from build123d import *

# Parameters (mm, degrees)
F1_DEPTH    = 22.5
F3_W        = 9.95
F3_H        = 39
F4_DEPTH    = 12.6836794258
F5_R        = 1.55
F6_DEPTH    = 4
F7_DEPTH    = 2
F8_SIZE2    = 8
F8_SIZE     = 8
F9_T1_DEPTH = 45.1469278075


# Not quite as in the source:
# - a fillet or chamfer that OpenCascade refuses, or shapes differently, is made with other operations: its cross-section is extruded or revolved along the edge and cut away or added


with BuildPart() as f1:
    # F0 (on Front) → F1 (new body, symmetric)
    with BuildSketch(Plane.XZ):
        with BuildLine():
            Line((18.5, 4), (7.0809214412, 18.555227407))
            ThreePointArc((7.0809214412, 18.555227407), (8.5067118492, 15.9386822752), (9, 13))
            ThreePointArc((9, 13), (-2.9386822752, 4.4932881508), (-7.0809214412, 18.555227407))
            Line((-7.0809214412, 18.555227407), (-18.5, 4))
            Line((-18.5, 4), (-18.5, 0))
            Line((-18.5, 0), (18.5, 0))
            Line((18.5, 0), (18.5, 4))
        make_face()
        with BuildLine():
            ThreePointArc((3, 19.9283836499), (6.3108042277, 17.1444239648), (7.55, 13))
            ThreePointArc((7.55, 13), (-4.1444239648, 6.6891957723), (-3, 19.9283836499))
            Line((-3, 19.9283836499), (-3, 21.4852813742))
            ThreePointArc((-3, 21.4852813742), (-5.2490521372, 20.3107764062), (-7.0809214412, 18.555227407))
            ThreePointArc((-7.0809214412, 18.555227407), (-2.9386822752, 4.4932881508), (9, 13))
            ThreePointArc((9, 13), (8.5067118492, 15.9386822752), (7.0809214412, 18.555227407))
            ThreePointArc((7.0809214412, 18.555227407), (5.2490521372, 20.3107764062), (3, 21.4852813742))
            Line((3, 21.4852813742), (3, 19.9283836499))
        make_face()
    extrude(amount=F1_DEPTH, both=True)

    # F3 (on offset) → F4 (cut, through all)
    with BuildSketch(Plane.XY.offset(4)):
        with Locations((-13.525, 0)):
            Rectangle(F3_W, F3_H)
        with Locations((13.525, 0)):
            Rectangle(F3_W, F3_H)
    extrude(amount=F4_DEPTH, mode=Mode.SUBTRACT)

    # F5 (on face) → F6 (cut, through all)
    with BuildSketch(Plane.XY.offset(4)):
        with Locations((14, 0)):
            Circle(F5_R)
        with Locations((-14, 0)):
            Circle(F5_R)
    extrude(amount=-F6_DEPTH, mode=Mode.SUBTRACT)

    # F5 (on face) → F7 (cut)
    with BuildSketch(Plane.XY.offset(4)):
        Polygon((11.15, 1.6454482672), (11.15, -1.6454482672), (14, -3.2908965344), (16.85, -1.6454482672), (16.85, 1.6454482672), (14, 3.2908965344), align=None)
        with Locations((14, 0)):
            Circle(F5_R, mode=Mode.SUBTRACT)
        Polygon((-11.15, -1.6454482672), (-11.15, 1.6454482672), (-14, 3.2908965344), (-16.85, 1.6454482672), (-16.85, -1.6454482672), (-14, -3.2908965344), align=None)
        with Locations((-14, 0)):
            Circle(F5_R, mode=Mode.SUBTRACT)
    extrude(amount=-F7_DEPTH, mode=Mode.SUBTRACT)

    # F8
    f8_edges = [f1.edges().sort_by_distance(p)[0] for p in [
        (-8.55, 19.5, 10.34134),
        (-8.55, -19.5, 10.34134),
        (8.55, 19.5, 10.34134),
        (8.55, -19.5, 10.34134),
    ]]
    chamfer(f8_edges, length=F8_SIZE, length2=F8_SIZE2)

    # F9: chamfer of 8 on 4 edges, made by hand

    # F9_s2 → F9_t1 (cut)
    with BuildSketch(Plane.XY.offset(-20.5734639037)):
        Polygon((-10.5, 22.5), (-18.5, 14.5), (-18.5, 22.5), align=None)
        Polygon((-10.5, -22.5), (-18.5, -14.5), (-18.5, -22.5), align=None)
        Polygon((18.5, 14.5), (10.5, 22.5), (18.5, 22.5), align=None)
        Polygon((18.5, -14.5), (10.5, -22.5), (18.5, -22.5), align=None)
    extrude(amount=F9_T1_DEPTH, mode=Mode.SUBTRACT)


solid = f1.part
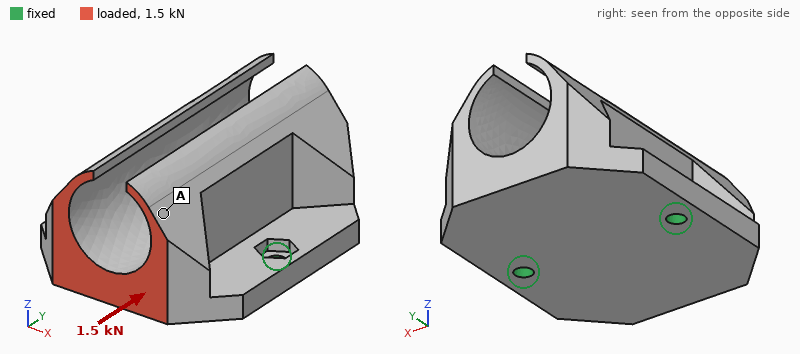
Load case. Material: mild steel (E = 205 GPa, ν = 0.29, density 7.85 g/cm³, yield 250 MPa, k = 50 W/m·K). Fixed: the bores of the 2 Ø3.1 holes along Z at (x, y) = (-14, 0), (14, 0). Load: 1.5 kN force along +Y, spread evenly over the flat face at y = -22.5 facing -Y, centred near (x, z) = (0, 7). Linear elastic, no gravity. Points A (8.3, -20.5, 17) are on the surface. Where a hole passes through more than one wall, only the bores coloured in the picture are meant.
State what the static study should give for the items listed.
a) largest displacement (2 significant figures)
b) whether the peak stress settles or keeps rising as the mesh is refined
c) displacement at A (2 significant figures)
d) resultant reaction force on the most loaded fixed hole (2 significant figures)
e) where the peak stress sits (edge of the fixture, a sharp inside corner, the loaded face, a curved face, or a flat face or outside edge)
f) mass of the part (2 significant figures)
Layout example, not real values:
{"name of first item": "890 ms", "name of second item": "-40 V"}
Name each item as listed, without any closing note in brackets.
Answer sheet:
{"largest displacement": "73 µm", "whether the peak stress settles or keeps rising as the mesh is refined": "keeps rising", "displacement at A": "63 µm", "resultant reaction force on the most loaded fixed hole": "750 N", "where the peak stress sits": "edge of the fixture", "mass of the part": "92 g"}
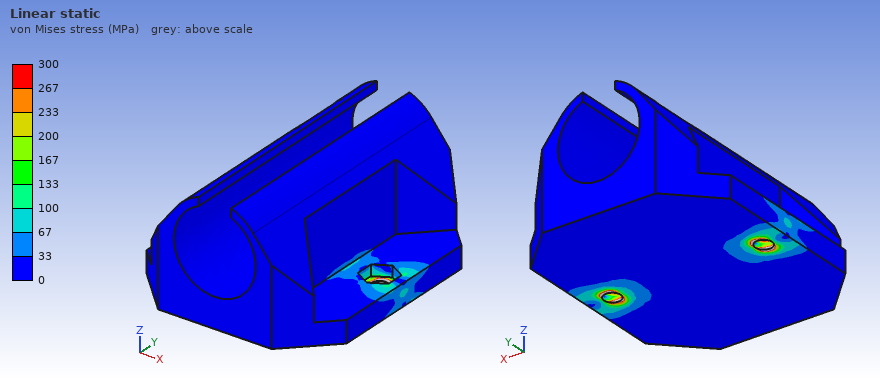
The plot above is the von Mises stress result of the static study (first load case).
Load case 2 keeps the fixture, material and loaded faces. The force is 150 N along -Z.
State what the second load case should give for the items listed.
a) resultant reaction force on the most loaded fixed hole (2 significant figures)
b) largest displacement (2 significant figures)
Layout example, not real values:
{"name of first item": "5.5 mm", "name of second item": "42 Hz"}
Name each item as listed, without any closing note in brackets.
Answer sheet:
{"resultant reaction force on the most loaded fixed hole": "96 N", "largest displacement": "29 µm"}
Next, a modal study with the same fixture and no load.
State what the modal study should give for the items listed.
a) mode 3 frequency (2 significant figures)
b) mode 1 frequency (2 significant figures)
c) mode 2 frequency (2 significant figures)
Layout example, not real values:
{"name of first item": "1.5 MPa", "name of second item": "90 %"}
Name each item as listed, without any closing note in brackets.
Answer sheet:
{"mode 3 frequency": "9000 Hz", "mode 1 frequency": "2100 Hz", "mode 2 frequency": "8700 Hz"}
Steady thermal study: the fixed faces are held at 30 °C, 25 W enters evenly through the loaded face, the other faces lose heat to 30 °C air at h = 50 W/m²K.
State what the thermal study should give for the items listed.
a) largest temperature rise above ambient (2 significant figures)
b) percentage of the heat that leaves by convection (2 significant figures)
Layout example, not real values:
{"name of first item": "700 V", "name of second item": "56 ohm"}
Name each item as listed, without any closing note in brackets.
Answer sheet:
{"largest temperature rise above ambient": "59 K", "percentage of the heat that leaves by convection": "35 %"}
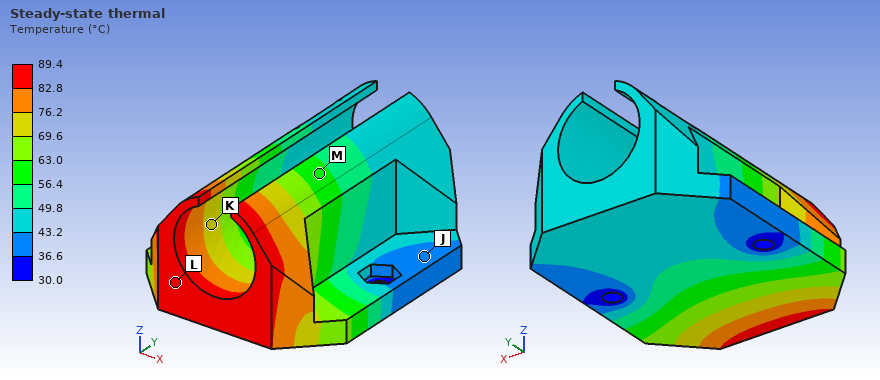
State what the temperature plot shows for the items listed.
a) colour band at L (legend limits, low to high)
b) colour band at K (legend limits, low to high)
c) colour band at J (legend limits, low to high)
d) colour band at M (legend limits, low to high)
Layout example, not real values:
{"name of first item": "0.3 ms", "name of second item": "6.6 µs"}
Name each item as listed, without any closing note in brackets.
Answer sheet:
{"colour band at L": "82.8 to 89.4 °C", "colour band at K": "69.6 to 76.2 °C", "colour band at J": "36.6 to 43.2 °C", "colour band at M": "56.4 to 63.0 °C"}
